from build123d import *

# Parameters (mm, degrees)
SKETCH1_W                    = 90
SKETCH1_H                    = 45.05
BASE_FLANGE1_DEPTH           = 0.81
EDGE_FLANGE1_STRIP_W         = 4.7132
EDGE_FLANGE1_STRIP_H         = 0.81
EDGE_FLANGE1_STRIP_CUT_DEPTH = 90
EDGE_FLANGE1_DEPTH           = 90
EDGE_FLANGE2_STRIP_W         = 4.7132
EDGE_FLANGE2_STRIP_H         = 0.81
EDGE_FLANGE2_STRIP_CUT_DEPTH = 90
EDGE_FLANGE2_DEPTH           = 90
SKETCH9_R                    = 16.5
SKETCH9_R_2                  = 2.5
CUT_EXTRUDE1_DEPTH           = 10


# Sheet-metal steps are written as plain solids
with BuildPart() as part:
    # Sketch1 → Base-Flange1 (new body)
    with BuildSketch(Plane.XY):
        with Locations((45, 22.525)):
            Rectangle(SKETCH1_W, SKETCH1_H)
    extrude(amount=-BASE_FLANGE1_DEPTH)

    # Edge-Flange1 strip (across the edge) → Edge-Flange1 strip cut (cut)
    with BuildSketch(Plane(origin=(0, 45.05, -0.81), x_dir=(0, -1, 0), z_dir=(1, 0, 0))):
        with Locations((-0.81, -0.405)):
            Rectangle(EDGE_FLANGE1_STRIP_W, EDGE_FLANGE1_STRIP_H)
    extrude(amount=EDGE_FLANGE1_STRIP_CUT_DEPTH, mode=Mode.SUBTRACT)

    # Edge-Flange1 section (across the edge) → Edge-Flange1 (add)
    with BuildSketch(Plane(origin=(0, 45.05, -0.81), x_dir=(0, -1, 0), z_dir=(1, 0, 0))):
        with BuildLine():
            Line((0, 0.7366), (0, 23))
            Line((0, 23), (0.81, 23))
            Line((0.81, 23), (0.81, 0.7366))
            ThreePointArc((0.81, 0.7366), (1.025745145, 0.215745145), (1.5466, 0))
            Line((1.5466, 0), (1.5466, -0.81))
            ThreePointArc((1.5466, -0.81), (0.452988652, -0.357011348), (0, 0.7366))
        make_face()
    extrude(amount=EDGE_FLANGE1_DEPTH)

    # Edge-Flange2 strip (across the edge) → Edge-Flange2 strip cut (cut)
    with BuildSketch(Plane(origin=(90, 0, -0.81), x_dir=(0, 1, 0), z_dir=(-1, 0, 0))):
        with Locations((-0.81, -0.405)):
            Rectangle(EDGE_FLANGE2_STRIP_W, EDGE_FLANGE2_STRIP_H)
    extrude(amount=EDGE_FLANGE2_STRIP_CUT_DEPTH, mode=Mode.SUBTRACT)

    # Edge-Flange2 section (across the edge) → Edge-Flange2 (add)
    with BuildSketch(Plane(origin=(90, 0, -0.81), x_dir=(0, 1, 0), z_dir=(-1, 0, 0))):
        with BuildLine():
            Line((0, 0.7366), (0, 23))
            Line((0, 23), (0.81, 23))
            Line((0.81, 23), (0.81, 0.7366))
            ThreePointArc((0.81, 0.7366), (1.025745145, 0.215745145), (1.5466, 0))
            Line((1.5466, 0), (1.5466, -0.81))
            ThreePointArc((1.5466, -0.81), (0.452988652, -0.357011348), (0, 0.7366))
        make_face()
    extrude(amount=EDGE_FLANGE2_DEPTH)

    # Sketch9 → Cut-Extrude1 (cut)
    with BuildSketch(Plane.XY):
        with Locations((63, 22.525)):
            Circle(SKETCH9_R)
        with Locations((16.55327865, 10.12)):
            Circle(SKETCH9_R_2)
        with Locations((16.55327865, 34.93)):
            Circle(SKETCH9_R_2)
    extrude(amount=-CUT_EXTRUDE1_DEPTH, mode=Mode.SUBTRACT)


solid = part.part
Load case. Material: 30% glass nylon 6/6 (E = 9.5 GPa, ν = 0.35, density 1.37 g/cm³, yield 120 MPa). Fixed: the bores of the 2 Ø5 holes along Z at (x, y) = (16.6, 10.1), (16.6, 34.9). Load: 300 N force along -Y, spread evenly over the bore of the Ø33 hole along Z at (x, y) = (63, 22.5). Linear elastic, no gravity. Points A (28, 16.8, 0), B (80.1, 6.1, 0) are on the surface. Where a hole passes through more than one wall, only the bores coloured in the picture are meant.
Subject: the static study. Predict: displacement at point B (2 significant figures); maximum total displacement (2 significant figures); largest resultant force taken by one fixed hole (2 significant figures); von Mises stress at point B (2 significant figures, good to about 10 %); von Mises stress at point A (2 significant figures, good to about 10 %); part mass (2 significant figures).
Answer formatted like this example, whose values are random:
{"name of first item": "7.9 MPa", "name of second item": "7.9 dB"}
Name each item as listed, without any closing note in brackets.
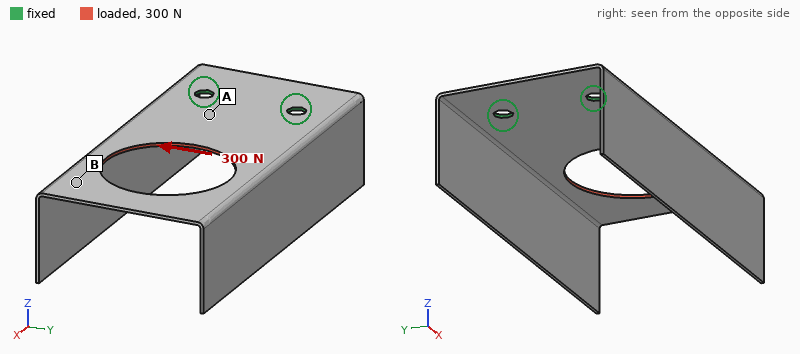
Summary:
{"displacement at point B": "0.85 mm", "maximum total displacement": "1.1 mm", "largest resultant force taken by one fixed hole": "520 N", "von Mises stress at point B": "12 MPa", "von Mises stress at point A": "29 MPa", "part mass": "8.0 g"}
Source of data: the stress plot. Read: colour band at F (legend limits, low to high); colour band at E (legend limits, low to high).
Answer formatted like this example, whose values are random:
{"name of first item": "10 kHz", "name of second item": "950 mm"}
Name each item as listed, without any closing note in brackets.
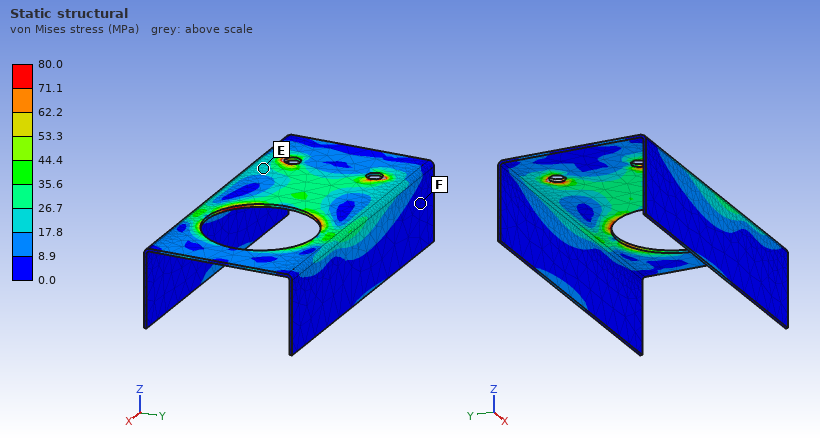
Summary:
{"colour band at F": "0.0 to 8.9 MPa", "colour band at E": "17.8 to 26.7 MPa"}
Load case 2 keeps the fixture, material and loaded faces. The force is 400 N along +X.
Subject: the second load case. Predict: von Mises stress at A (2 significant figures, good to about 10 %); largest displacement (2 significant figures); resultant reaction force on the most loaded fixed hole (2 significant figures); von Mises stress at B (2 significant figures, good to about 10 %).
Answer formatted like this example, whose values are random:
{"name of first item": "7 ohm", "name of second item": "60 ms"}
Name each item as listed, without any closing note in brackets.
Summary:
{"von Mises stress at A": "6.4 MPa", "largest displacement": "0.26 mm", "resultant reaction force on the most loaded fixed hole": "200 N", "von Mises stress at B": "7.3 MPa"}
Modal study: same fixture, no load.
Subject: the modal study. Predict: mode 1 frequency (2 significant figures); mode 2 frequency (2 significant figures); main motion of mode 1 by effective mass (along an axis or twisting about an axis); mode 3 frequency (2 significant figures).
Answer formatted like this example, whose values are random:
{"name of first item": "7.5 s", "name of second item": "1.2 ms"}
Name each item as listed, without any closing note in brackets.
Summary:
{"mode 1 frequency": "130 Hz", "mode 2 frequency": "150 Hz", "main motion of mode 1 by effective mass": "along Z", "mode 3 frequency": "270 Hz"}
